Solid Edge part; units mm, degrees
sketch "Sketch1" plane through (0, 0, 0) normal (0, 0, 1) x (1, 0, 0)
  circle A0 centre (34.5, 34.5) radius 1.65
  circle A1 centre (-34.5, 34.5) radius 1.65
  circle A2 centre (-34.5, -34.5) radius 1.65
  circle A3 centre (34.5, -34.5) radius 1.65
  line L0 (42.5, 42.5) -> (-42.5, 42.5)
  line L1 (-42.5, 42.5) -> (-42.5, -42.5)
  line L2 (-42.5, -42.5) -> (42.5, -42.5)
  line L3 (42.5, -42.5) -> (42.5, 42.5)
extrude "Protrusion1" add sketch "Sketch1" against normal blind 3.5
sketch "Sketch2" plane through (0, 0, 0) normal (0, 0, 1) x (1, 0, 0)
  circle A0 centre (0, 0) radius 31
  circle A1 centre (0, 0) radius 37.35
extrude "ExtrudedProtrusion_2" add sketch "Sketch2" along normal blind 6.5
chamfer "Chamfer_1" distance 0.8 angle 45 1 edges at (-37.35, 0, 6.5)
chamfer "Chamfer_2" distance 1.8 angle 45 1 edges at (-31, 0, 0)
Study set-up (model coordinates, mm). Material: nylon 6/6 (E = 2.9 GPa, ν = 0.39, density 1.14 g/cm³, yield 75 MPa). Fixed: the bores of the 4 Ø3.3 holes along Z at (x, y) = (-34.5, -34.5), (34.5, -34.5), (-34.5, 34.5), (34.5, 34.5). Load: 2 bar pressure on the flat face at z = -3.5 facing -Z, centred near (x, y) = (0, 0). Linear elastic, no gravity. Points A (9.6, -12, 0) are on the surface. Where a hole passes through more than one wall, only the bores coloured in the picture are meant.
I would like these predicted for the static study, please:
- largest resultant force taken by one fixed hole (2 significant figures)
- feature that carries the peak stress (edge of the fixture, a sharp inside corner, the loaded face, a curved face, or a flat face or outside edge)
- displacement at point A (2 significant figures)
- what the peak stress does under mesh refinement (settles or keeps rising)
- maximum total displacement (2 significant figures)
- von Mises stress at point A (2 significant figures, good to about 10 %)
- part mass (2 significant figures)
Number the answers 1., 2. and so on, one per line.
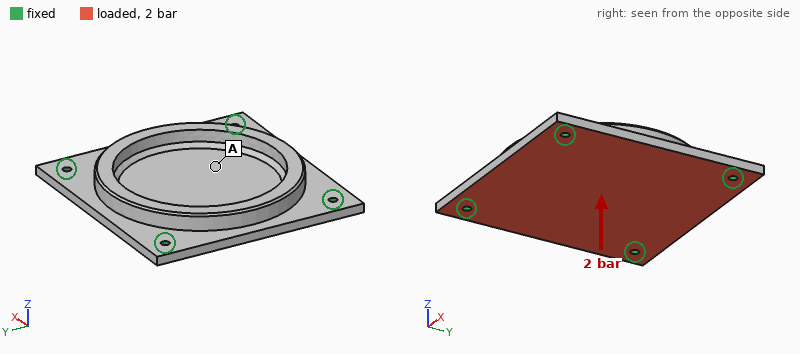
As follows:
1. 400 N
2. edge of the fixture
3. 1.1 mm
4. keeps rising
5. 1.2 mm
6. 8.2 MPa
7. 39 g
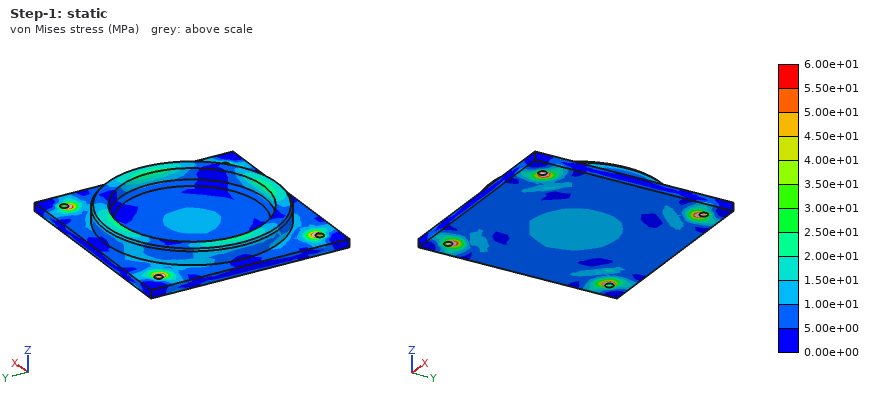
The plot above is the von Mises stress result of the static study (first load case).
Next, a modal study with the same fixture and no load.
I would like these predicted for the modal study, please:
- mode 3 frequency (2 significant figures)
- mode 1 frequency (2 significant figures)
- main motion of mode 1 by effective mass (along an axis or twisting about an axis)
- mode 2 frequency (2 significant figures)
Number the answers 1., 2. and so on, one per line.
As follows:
1. 1600 Hz
2. 1100 Hz
3. along Z
4. 1600 Hz
